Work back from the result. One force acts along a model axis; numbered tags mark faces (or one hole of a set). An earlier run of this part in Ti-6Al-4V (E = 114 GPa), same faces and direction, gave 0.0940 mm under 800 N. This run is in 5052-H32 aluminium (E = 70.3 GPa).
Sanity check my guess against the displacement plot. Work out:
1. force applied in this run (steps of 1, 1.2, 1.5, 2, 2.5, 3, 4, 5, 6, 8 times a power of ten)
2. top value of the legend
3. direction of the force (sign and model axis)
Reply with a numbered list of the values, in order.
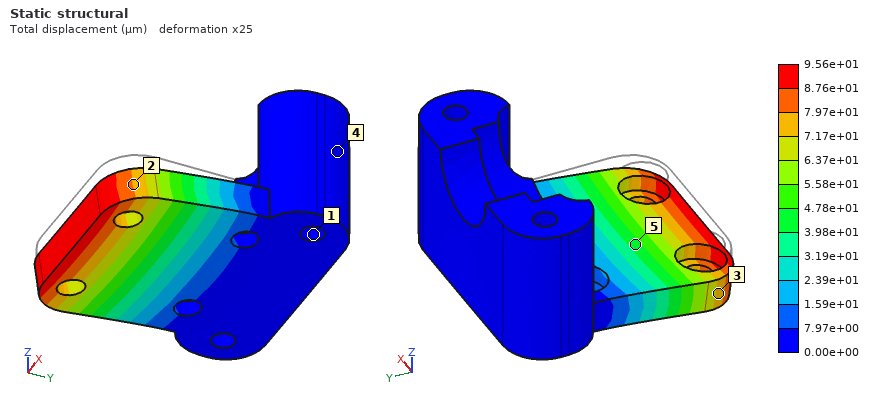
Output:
1. 500 N
2. 9.56e+01 µm
3. -Z
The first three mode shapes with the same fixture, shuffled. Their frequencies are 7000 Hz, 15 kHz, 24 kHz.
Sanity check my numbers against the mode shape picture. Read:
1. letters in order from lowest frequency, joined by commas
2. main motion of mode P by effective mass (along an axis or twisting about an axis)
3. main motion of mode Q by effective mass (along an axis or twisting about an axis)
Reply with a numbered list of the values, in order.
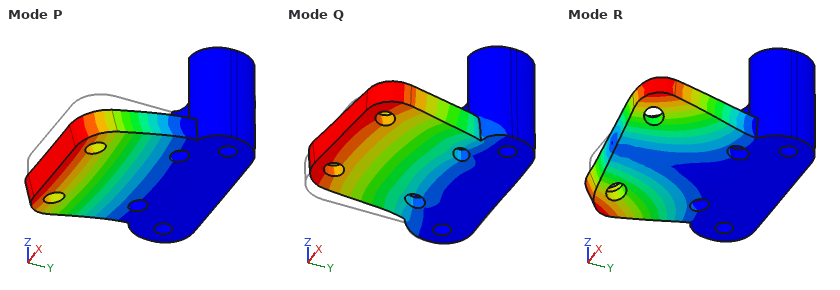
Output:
1. P, R, Q
2. along Z
3. along X
